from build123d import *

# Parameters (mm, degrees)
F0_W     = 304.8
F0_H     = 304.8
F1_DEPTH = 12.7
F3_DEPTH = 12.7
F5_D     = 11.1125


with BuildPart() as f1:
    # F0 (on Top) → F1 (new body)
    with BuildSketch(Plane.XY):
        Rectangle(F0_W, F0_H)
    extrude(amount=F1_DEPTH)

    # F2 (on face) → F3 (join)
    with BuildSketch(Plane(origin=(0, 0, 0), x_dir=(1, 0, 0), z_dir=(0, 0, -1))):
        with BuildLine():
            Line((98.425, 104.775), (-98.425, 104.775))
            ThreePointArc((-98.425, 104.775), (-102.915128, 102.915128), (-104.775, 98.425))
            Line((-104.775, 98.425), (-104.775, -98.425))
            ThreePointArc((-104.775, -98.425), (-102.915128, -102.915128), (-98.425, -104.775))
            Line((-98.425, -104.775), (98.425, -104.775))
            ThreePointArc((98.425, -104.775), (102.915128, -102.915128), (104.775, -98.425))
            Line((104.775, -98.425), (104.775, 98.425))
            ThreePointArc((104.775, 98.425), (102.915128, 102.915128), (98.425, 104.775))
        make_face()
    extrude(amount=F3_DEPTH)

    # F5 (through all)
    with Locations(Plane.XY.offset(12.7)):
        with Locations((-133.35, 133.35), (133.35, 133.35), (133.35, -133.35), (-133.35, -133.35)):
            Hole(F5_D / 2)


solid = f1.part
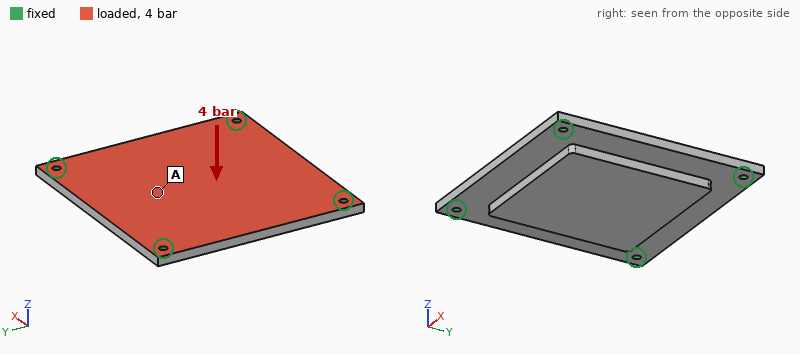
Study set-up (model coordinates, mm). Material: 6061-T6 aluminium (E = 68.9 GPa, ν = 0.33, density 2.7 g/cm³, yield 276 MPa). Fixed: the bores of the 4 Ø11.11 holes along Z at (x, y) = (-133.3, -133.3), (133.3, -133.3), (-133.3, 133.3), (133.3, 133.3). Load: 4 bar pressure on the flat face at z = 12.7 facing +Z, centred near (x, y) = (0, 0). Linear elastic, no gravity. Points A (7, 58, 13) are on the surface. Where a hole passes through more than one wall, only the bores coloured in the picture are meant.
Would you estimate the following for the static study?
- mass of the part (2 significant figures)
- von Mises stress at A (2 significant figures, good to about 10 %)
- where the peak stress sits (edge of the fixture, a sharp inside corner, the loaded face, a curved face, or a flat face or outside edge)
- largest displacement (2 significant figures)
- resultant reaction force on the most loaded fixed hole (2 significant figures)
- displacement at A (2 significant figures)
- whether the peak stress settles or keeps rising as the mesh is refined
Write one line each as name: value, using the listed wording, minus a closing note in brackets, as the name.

mass of the part: 4.7 kg
von Mises stress at A: 18 MPa
where the peak stress sits: edge of the fixture
largest displacement: 0.44 mm
resultant reaction force on the most loaded fixed hole: 12 kN
displacement at A: 0.41 mm
whether the peak stress settles or keeps rising as the mesh is refined: keeps rising
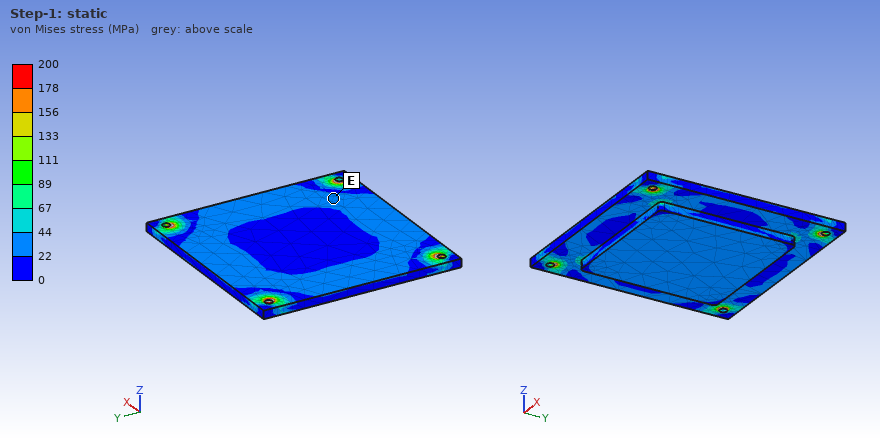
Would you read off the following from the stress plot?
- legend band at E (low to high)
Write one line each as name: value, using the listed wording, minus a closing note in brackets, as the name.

legend band at E: 22 to 44 MPa
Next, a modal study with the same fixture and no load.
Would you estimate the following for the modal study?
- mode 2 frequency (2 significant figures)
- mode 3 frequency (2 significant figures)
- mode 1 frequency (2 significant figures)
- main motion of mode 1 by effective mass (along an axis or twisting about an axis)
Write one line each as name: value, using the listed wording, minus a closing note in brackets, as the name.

mode 2 frequency: 1200 Hz
mode 3 frequency: 1200 Hz
mode 1 frequency: 710 Hz
main motion of mode 1 by effective mass: along Z
